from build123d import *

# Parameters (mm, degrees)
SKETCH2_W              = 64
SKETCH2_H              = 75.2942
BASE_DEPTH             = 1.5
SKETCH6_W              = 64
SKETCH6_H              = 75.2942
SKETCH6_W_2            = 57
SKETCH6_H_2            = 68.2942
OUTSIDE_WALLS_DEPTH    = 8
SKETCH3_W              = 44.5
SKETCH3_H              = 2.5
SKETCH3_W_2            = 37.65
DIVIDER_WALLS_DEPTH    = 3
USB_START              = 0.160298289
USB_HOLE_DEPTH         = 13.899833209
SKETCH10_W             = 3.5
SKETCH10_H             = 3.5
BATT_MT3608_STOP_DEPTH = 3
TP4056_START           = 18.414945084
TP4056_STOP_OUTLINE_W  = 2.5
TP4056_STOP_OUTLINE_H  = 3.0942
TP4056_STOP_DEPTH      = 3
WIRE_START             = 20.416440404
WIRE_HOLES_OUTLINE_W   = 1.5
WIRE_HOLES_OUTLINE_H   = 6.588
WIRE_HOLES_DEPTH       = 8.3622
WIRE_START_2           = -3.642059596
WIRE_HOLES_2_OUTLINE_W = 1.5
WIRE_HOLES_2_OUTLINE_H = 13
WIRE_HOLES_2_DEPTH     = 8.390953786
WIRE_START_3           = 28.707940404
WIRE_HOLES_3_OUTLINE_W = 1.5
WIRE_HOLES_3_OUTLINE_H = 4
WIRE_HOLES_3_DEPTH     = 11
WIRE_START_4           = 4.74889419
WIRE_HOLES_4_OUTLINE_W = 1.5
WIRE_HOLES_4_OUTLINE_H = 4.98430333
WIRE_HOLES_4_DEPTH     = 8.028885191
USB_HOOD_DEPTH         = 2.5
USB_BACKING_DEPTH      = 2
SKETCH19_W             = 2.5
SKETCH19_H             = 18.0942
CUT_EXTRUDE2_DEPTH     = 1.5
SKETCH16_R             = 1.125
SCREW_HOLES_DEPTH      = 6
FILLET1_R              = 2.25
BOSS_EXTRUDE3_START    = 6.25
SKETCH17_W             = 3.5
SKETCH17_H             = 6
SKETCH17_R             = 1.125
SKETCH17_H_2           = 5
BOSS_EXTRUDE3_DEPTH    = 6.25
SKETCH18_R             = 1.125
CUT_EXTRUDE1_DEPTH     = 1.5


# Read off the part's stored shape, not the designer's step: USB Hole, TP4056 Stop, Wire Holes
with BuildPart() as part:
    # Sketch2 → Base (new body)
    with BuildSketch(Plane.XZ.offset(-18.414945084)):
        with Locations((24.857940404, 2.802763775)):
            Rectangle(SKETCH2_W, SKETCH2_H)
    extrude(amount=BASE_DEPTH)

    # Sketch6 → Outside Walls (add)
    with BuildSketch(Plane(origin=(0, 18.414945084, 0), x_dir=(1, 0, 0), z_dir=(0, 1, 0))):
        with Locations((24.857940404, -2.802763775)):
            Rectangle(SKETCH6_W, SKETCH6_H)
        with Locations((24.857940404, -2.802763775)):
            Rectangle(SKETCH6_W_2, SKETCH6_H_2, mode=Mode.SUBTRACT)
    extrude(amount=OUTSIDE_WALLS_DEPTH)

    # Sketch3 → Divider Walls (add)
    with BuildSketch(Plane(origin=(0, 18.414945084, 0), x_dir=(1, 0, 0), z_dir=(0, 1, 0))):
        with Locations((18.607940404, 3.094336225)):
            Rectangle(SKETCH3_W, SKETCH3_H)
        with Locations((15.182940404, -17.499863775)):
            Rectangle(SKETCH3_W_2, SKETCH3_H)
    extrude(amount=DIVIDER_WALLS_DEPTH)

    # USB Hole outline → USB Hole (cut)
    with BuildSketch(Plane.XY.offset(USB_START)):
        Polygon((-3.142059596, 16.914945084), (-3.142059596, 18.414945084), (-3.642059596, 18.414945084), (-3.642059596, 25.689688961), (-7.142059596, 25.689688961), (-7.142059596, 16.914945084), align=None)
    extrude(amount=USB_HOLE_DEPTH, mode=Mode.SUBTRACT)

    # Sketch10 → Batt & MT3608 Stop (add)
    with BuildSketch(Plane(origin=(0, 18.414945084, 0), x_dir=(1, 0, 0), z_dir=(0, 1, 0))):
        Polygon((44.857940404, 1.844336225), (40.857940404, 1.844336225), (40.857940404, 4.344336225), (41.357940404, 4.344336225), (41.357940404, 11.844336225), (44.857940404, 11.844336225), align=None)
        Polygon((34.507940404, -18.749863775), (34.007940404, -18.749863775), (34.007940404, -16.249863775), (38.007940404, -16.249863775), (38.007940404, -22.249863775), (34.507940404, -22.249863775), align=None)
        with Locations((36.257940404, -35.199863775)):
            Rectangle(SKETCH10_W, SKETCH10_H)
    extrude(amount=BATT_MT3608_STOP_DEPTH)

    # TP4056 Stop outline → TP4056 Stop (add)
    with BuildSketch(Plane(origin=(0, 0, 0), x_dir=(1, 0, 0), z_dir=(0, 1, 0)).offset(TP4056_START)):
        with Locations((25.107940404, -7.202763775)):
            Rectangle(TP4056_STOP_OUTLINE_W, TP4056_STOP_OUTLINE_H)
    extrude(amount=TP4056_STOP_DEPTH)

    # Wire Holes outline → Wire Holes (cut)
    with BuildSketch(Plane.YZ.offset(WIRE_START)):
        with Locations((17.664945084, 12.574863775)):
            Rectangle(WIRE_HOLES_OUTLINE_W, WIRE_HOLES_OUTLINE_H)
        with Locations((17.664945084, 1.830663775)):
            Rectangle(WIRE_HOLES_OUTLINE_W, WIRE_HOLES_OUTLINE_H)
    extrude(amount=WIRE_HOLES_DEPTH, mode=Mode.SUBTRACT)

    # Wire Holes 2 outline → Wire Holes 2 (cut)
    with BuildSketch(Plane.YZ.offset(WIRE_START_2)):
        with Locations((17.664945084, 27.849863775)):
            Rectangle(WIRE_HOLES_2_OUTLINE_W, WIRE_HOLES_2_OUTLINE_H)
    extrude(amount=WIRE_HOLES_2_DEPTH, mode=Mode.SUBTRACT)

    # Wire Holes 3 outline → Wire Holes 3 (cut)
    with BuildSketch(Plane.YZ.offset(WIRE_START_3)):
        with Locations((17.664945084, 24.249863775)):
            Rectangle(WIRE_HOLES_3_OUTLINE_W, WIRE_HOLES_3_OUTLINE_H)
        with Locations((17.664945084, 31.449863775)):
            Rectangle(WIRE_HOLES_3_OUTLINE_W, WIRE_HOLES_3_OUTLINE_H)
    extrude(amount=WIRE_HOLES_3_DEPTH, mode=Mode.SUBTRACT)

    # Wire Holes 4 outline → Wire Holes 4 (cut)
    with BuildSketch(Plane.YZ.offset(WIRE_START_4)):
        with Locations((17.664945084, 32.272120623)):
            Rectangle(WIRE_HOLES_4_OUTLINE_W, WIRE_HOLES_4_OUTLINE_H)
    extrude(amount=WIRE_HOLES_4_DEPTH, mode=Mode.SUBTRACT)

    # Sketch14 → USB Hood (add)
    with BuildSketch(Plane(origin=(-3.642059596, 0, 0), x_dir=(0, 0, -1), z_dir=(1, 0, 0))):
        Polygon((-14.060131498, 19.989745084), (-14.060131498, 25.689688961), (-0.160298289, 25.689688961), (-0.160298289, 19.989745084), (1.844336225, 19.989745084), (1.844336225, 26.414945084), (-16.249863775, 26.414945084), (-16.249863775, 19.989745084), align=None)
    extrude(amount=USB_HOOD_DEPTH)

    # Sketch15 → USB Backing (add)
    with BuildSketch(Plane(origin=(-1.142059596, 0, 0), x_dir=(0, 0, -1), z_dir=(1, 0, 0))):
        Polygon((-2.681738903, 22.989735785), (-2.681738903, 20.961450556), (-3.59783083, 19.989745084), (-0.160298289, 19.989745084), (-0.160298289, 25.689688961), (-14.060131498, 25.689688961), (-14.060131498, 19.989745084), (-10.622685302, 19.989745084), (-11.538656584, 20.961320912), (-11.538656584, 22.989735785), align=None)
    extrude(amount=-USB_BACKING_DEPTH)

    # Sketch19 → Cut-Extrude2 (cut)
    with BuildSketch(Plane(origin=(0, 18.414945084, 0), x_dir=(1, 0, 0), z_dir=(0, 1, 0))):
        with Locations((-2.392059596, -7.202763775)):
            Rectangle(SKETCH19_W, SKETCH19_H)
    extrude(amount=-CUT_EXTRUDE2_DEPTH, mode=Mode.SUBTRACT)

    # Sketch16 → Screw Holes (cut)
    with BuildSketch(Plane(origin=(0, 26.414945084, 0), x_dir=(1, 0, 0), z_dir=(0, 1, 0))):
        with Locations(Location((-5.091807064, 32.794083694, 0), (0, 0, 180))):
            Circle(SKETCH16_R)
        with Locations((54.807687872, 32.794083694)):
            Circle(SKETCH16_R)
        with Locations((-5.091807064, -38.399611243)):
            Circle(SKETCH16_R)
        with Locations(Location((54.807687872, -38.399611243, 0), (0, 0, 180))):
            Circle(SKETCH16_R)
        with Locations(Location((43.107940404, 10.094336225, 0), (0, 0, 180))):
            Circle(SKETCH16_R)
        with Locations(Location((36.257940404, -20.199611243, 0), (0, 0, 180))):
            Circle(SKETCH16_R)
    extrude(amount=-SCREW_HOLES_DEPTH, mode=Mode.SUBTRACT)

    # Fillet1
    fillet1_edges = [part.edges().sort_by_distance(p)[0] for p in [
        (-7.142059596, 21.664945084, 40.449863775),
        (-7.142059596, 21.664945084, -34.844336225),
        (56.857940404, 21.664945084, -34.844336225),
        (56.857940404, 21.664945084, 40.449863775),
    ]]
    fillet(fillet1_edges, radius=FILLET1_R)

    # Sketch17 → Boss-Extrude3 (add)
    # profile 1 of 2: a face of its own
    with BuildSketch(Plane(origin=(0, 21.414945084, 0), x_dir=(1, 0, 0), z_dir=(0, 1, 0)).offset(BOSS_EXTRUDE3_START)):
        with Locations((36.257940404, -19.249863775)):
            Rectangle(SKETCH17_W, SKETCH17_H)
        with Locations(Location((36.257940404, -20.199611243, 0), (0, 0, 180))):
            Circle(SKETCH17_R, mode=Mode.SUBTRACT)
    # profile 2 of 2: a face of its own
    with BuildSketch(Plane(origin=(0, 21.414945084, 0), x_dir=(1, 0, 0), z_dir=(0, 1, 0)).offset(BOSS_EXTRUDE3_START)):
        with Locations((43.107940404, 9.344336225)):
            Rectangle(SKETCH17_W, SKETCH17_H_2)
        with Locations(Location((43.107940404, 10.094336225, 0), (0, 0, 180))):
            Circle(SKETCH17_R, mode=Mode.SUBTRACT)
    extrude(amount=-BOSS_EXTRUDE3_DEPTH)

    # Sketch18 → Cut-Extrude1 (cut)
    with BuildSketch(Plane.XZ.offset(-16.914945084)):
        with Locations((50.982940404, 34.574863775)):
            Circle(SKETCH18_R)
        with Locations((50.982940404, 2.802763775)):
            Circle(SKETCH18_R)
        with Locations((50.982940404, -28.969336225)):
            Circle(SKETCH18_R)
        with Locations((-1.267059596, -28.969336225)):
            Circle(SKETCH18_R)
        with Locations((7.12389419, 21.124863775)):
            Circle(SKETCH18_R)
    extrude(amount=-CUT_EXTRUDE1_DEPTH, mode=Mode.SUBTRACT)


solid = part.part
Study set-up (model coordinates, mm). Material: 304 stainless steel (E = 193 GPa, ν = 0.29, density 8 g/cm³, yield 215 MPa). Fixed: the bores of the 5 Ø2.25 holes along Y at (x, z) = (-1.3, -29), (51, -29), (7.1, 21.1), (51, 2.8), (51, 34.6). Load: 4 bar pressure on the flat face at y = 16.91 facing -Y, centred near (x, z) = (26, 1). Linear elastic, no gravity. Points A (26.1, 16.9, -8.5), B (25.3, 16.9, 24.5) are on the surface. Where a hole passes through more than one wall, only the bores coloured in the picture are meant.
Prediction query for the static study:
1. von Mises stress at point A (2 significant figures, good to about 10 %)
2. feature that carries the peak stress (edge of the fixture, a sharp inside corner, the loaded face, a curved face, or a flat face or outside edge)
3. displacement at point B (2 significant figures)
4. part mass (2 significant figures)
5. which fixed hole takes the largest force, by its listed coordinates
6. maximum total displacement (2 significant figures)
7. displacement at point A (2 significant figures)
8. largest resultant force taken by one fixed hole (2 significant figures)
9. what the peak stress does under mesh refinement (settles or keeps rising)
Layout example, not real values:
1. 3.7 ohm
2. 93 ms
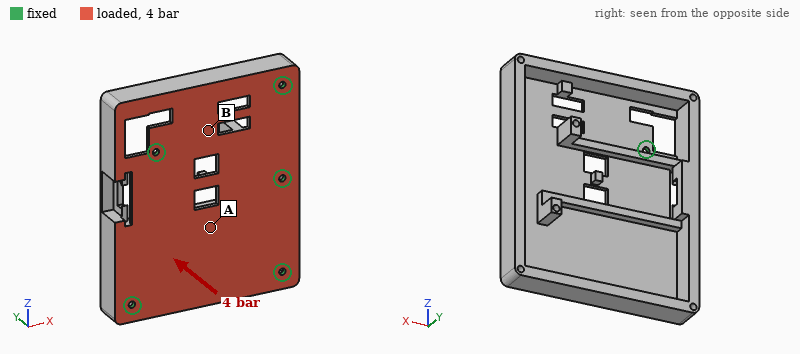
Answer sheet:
1. 45 MPa
2. edge of the fixture
3. 25 µm
4. 120 g
5. (7.1, 21.1)
6. 62 µm
7. 61 µm
8. 560 N
9. keeps rising
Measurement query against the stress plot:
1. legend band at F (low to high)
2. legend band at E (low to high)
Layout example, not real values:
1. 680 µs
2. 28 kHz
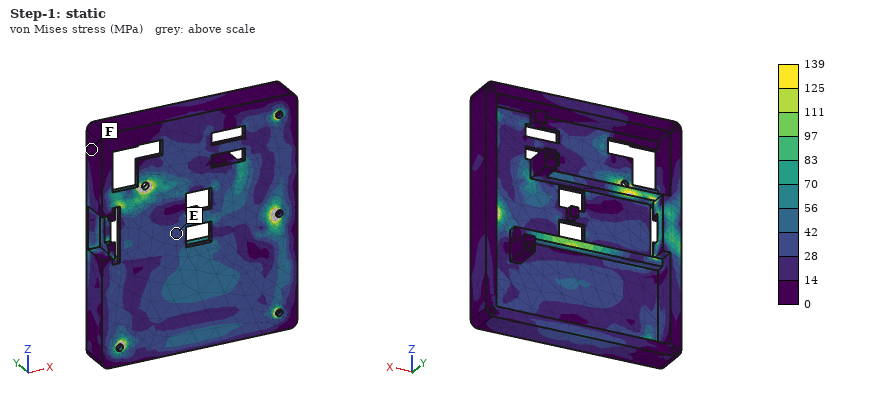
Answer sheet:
1. 0 to 14 MPa
2. 28 to 42 MPa
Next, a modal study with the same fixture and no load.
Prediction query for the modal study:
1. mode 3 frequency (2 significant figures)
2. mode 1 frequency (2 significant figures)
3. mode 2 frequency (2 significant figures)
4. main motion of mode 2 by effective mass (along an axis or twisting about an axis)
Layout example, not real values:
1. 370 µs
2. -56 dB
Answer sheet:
1. 5100 Hz
2. 2700 Hz
3. 3900 Hz
4. along Y
